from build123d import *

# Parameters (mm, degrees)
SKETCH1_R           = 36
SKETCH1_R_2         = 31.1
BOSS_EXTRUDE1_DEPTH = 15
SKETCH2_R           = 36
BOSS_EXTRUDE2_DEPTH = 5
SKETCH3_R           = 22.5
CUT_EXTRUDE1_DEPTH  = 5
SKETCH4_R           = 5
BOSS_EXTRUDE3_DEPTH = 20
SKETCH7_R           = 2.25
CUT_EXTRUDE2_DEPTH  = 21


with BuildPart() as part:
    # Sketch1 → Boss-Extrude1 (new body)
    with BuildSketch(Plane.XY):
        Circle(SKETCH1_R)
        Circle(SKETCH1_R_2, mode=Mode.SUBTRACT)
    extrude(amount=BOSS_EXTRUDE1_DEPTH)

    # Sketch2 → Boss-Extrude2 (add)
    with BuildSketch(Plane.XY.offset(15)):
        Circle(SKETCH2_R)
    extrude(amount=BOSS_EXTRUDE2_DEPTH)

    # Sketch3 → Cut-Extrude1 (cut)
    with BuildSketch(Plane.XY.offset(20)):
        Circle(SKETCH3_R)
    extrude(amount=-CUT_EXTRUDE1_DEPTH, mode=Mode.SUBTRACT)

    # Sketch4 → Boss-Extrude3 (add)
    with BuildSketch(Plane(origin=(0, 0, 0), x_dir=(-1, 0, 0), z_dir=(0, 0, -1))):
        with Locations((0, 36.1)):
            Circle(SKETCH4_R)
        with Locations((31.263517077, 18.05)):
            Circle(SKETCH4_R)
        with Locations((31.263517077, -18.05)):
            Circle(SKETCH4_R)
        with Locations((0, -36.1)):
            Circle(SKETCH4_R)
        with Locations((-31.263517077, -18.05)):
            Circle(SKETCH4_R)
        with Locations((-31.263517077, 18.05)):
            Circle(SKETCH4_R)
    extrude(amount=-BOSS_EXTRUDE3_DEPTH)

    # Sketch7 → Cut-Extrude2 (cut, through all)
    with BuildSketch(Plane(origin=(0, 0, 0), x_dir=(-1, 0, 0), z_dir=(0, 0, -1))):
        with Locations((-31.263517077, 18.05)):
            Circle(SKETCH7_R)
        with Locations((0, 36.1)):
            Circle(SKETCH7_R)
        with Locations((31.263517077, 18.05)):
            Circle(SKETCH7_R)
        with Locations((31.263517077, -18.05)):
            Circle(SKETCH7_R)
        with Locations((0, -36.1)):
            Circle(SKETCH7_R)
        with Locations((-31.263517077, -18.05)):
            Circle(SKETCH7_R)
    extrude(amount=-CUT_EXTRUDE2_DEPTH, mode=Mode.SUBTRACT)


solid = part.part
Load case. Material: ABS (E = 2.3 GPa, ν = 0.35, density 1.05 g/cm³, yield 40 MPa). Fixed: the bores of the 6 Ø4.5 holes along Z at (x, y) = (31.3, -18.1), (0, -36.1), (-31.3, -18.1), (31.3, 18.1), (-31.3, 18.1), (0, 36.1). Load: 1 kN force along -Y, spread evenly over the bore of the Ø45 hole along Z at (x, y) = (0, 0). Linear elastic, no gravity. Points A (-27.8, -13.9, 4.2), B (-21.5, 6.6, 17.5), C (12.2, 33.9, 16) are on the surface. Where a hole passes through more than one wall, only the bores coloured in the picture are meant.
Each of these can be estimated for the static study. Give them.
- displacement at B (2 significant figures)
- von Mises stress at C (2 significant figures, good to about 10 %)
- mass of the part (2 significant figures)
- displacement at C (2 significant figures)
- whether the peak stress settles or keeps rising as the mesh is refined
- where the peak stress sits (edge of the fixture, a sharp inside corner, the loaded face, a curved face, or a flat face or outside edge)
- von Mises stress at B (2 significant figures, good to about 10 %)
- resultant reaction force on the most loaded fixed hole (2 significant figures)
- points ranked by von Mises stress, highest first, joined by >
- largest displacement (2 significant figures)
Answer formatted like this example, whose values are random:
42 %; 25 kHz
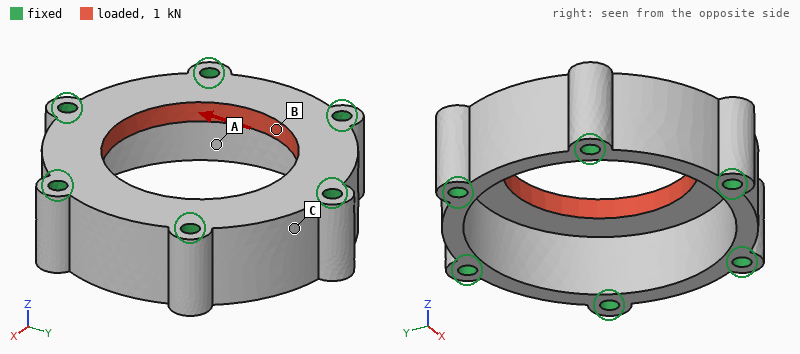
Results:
16 µm; 0.97 MPa; 33 g; 15 µm; keeps rising; edge of the fixture; 2.7 MPa; 210 N; B > C > A; 29 µm
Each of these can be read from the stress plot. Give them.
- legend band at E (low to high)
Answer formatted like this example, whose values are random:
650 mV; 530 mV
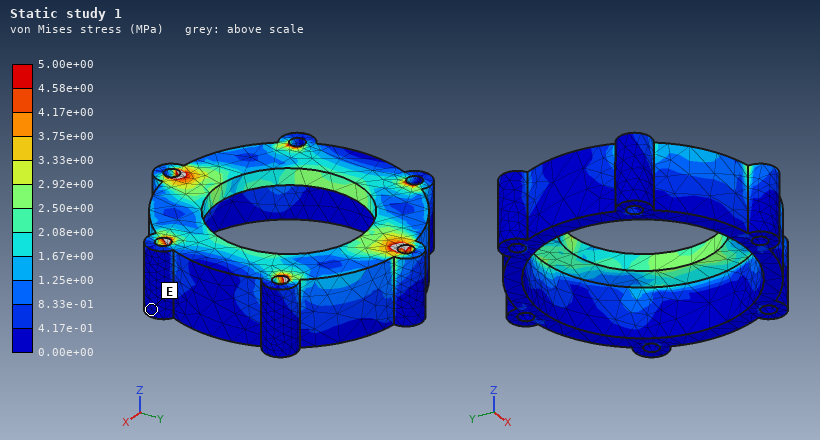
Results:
0.00e+00 to 4.17e-01 MPa
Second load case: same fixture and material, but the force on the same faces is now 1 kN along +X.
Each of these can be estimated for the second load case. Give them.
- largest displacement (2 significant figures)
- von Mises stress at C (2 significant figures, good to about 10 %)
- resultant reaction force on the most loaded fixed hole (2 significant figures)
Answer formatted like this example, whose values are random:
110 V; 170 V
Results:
32 µm; 0.84 MPa; 190 N
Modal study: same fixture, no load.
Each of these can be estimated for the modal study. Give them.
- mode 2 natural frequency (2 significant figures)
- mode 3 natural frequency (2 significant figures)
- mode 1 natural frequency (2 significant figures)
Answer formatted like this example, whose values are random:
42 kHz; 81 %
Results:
7800 Hz; 8100 Hz; 7700 Hz
